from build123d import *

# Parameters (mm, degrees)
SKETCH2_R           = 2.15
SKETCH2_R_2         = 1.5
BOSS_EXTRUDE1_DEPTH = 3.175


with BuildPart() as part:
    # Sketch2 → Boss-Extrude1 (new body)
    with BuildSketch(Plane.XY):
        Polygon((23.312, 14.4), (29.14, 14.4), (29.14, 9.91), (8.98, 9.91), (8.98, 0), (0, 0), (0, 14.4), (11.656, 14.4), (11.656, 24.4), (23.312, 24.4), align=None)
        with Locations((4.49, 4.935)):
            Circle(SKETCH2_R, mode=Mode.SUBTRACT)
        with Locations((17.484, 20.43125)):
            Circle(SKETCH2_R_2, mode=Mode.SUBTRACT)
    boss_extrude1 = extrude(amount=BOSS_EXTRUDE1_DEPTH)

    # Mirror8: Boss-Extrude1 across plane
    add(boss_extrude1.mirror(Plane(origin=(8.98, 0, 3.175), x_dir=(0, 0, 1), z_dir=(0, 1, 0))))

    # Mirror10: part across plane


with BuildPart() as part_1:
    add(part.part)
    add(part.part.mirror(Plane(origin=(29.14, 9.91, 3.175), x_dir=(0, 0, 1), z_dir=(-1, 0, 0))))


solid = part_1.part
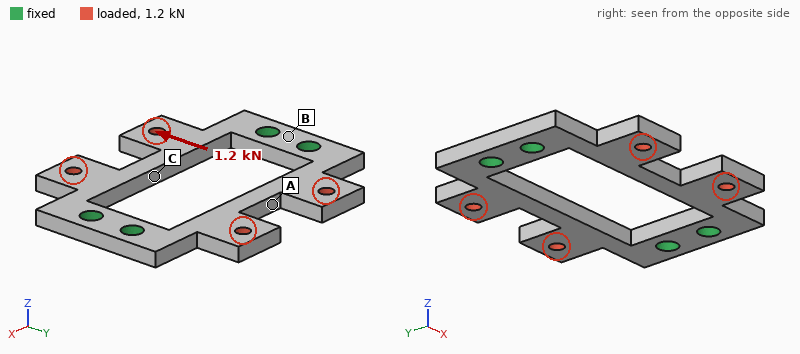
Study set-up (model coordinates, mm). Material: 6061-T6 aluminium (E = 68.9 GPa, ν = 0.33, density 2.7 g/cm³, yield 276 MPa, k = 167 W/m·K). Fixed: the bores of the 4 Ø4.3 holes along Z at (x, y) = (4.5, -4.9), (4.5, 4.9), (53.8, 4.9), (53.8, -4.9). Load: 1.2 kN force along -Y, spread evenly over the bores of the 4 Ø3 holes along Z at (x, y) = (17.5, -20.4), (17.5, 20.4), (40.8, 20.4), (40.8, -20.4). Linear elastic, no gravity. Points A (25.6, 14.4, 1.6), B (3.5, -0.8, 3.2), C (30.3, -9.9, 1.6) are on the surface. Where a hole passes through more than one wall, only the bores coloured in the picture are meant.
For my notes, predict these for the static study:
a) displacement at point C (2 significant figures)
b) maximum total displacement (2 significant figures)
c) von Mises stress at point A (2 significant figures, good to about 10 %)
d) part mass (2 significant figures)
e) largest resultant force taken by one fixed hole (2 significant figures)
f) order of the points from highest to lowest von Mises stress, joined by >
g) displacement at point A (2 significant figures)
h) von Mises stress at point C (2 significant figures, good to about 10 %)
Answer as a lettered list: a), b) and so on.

a) 0.092 mm
b) 0.11 mm
c) 120 MPa
d) 11 g
e) 350 N
f) A > C > B
g) 0.088 mm
h) 86 MPa
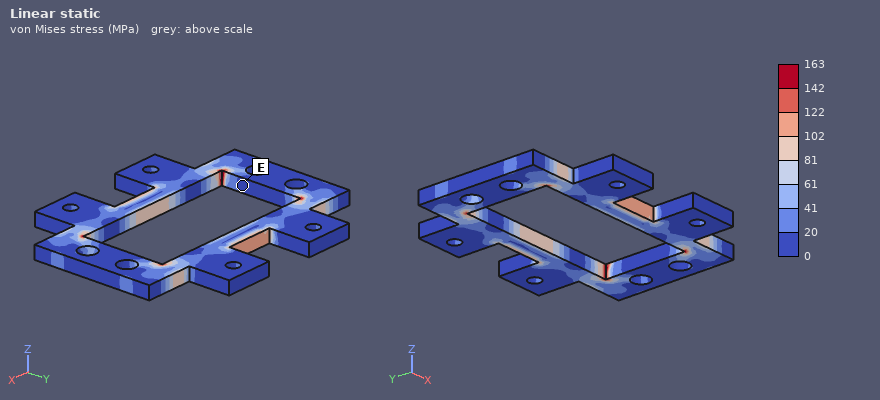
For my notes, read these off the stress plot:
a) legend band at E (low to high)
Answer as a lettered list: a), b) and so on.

a) 0 to 20 MPa
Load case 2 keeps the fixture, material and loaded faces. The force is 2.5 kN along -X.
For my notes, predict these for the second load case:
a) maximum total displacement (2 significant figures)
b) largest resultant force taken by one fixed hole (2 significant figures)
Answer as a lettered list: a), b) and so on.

a) 49 µm
b) 670 N
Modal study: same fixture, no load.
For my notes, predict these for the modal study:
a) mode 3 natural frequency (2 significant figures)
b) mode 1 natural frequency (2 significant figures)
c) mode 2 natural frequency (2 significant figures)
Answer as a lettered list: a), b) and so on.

a) 6600 Hz
b) 3700 Hz
c) 3700 Hz
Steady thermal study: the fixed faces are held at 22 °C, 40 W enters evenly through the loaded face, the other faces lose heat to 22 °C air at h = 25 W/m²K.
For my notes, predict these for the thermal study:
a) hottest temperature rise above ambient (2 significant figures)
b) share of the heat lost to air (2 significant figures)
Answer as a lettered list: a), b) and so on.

a) 55 K
b) 6.9 %
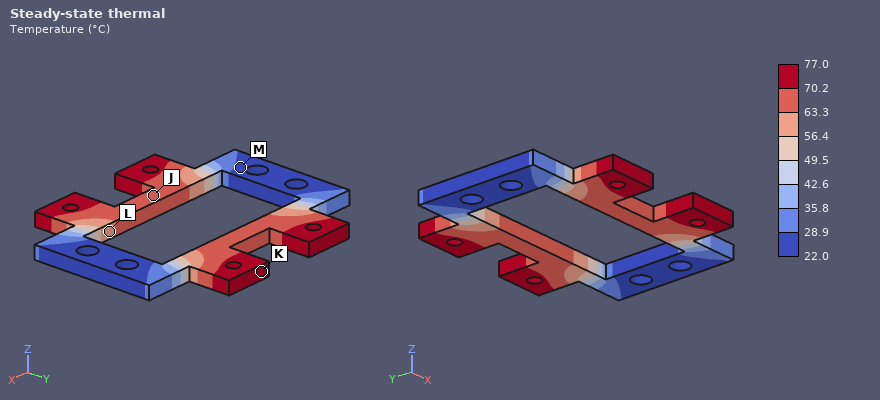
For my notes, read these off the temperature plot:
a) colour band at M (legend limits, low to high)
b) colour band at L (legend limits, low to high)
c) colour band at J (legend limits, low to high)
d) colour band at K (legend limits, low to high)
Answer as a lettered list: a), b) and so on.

a) 22.0 to 28.9 °C
b) 56.4 to 63.3 °C
c) 63.3 to 70.2 °C
d) 70.2 to 77.0 °C
